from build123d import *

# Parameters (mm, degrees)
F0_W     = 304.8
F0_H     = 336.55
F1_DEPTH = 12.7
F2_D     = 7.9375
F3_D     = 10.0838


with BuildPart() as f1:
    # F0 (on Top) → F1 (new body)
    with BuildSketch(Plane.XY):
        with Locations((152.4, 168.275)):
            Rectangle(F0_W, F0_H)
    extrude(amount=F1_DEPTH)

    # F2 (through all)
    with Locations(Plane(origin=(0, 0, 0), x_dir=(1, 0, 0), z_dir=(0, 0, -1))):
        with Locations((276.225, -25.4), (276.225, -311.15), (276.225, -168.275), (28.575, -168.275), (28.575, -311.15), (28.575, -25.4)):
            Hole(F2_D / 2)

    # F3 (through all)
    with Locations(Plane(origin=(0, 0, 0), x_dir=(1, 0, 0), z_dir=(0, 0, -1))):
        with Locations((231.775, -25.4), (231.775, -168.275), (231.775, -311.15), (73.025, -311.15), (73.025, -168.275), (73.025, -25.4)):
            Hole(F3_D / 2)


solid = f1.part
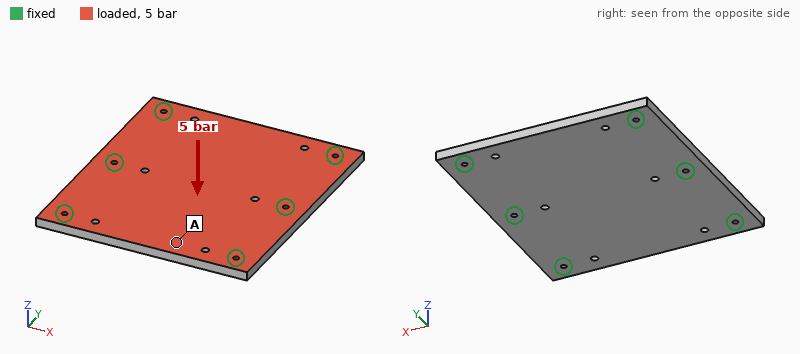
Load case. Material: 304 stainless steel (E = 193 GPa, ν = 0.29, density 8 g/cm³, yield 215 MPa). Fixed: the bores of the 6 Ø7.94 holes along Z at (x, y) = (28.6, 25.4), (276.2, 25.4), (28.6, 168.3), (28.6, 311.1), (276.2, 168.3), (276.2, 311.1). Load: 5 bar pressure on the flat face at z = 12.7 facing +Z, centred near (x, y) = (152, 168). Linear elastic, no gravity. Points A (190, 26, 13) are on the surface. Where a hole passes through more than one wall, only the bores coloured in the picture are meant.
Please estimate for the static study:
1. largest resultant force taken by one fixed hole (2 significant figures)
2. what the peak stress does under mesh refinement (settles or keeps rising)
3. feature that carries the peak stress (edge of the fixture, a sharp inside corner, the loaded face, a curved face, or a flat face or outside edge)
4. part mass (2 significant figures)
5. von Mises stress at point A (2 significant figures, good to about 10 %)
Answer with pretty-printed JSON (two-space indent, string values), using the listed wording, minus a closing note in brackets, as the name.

{
  "largest resultant force taken by one fixed hole": "11 kN",
  "what the peak stress does under mesh refinement": "keeps rising",
  "feature that carries the peak stress": "edge of the fixture",
  "part mass": "10 kg",
  "von Mises stress at point A": "45 MPa"
}
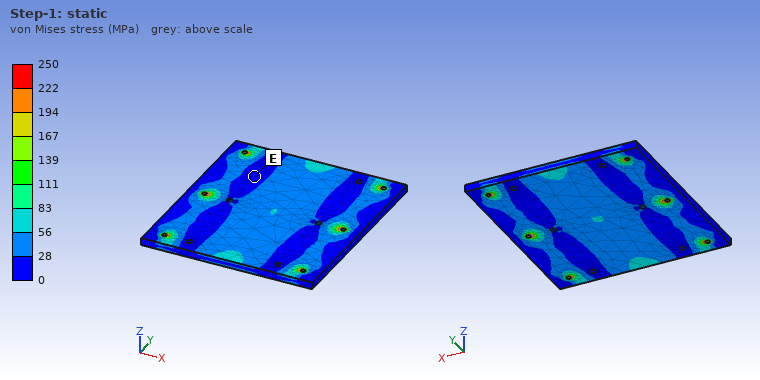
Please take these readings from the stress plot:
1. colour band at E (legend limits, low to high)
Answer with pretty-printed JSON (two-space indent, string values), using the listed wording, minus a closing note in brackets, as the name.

{
  "colour band at E": "0 to 28 MPa"
}
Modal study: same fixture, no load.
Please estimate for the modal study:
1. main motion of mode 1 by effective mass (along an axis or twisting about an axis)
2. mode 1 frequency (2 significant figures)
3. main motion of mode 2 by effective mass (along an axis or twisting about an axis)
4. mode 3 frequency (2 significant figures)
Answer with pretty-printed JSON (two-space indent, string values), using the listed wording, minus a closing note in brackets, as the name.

{
  "main motion of mode 1 by effective mass": "along Z",
  "mode 1 frequency": "830 Hz",
  "main motion of mode 2 by effective mass": "twisting about X",
  "mode 3 frequency": "1500 Hz"
}
